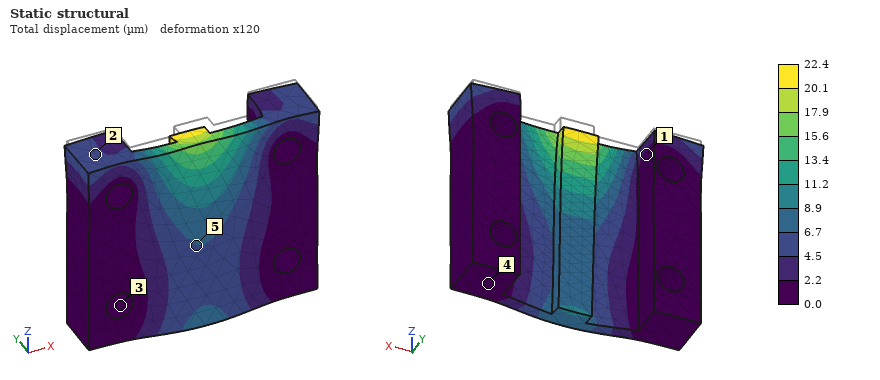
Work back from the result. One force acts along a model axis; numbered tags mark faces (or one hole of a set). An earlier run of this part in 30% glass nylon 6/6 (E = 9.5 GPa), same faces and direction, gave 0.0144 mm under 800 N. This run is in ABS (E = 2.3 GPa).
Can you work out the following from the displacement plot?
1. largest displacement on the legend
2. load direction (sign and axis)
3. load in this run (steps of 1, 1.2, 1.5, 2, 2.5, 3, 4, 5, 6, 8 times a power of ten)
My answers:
22.4 µm
-Z
300 N
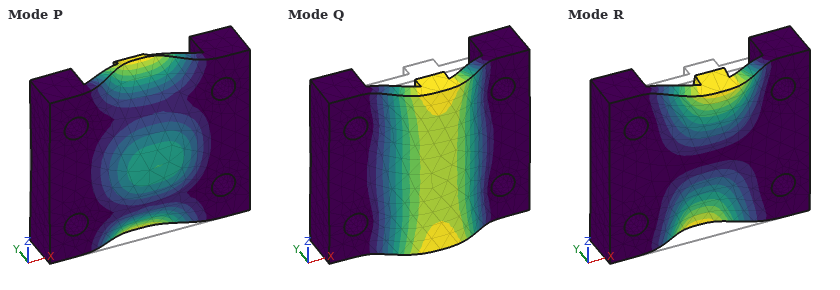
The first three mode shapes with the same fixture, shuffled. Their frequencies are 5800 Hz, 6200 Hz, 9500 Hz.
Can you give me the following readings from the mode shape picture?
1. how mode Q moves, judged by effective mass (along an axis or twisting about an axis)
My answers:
along Y
